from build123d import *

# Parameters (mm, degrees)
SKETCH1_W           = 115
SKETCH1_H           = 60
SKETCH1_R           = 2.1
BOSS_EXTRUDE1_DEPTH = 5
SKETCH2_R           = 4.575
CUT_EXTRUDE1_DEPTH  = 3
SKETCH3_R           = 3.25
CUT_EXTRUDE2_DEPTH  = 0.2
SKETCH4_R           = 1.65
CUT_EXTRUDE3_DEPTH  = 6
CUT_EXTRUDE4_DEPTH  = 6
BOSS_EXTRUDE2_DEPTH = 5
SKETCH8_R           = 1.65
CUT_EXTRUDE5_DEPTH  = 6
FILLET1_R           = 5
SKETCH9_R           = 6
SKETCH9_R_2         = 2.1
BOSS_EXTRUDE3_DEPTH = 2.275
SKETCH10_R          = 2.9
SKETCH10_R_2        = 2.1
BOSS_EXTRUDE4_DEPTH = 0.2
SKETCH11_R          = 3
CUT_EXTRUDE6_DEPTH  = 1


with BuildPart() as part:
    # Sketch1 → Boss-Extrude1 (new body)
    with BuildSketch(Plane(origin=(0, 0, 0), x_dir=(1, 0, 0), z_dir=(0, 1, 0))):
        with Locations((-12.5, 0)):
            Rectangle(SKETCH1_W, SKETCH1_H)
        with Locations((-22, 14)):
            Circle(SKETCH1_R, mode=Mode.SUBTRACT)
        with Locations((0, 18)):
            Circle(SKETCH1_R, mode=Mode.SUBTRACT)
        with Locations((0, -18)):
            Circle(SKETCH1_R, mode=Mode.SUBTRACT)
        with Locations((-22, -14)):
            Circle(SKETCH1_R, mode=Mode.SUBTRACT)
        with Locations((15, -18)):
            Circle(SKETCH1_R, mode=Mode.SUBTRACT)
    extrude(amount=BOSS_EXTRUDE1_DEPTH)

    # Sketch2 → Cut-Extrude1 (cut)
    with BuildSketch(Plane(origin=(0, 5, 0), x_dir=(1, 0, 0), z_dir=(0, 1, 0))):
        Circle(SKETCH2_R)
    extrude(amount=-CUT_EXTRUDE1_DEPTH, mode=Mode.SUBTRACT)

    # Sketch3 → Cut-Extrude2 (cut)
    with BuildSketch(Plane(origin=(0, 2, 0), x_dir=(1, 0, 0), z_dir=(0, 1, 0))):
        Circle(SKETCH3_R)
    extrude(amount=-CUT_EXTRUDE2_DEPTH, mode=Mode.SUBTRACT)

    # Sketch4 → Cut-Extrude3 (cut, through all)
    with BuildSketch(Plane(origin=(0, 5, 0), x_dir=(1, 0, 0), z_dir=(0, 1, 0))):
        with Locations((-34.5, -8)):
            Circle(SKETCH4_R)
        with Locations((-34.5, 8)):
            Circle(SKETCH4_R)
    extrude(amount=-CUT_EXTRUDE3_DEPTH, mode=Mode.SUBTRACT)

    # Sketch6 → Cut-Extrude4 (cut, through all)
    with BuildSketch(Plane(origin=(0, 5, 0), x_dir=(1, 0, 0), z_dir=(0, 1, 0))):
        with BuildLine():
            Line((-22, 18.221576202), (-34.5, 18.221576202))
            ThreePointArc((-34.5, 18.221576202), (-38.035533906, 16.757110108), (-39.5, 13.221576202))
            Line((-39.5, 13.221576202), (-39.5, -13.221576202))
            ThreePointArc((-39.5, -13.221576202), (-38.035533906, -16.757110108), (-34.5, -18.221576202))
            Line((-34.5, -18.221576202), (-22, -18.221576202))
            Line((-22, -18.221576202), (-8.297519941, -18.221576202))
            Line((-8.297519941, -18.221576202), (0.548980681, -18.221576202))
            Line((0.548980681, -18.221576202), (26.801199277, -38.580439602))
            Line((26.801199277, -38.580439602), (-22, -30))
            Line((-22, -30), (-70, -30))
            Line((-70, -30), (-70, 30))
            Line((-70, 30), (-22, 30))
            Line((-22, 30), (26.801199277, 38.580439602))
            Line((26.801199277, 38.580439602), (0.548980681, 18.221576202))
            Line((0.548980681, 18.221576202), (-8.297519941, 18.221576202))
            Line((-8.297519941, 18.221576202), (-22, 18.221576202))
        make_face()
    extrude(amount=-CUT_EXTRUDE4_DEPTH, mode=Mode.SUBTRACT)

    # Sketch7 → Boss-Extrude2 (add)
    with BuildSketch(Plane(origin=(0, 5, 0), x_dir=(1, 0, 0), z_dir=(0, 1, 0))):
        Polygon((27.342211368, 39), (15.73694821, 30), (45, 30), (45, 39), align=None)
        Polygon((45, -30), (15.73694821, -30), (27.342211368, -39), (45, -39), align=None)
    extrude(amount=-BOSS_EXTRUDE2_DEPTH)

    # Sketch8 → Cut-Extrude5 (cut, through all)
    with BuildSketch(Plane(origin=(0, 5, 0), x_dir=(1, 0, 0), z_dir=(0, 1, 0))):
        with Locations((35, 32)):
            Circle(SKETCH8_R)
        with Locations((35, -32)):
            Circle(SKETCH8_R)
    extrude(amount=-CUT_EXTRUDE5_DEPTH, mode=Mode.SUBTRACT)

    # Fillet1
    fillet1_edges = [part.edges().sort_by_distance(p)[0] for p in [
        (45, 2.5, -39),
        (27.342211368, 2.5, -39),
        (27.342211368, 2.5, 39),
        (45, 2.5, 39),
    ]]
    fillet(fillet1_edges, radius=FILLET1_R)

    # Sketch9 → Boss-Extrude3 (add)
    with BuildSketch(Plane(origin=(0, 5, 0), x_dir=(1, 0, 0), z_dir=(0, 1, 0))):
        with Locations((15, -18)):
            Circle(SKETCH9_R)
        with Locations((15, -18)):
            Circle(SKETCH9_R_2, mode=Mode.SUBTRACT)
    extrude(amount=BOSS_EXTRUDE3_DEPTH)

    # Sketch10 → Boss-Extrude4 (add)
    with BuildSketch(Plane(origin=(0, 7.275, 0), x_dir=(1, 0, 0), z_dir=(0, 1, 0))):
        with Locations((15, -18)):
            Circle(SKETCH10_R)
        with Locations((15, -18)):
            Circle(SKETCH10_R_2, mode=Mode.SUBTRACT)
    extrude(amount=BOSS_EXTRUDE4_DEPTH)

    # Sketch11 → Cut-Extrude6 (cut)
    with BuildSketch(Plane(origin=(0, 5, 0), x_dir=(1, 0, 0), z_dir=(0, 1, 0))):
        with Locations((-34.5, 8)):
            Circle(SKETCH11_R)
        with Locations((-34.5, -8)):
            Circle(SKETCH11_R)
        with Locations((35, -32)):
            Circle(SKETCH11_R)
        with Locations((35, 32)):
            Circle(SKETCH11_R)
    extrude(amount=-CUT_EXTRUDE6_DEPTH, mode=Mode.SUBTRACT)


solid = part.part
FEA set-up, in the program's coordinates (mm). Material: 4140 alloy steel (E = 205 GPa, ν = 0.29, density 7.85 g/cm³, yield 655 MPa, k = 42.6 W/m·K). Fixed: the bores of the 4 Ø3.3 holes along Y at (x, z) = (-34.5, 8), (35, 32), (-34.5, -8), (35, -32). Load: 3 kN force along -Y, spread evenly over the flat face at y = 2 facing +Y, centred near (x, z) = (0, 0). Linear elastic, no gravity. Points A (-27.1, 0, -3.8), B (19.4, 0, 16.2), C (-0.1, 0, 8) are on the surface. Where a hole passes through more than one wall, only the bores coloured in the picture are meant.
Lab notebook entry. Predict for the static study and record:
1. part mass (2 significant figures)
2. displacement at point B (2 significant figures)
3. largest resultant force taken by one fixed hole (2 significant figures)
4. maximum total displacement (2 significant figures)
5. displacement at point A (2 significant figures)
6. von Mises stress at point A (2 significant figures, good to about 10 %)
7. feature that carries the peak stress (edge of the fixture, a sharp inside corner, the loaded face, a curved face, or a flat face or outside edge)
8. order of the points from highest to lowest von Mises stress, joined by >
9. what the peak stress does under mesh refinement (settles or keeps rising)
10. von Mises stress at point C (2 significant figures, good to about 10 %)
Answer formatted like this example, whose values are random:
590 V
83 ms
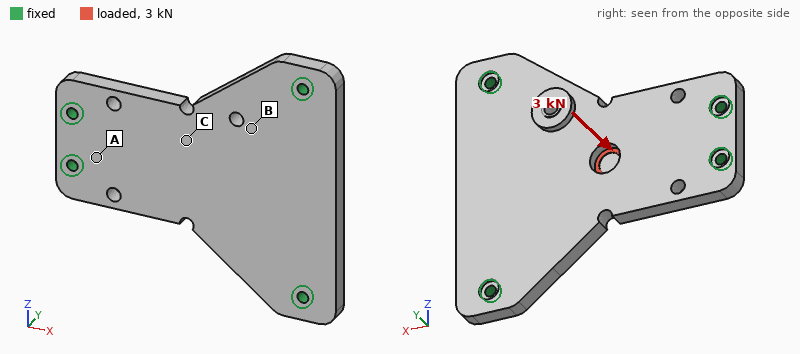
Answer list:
170 g
0.057 mm
810 N
0.11 mm
0.018 mm
99 MPa
edge of the fixture
C > A > B
keeps rising
180 MPa
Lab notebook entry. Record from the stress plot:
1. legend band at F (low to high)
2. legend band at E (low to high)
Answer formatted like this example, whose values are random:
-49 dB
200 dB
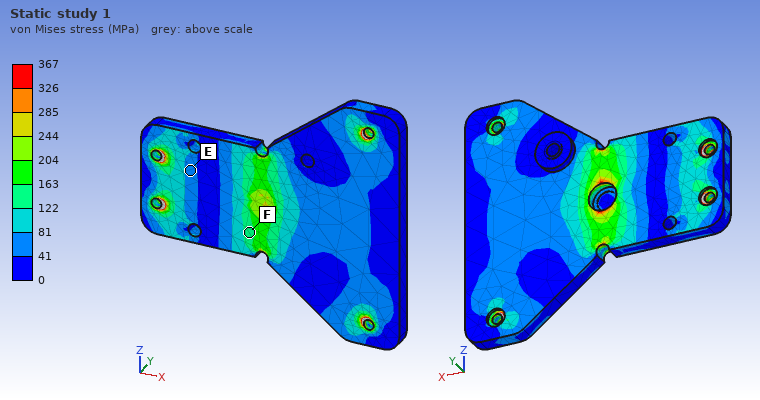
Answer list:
122 to 163 MPa
41 to 81 MPa
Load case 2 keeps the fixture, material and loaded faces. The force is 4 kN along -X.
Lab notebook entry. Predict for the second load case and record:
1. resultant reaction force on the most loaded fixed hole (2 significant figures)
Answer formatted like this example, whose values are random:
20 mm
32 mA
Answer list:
1.2 kN
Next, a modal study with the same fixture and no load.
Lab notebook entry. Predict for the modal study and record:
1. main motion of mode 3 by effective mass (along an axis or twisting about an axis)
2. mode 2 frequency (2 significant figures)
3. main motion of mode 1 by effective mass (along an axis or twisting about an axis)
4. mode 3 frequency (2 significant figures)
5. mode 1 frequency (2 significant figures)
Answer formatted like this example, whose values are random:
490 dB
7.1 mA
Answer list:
twisting about X
6200 Hz
along Y
7200 Hz
3800 Hz
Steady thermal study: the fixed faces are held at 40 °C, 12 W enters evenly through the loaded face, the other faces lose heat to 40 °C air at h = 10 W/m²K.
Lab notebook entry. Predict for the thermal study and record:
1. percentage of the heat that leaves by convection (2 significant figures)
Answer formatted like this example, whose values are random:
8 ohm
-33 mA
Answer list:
9.8 %
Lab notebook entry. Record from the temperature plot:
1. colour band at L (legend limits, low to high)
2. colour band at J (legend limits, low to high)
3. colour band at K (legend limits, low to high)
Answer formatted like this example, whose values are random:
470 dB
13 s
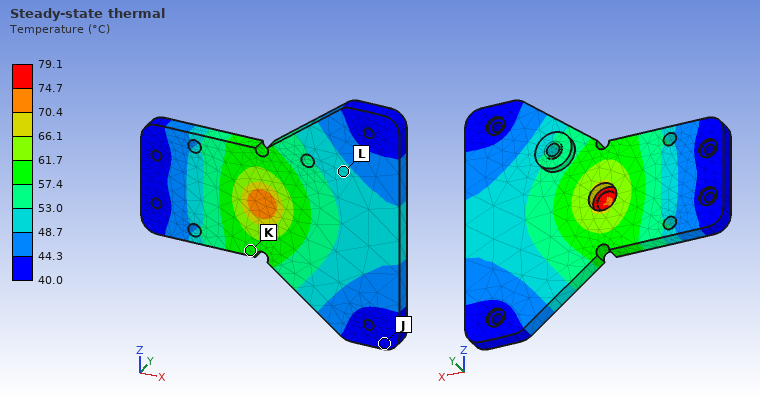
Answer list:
48.7 to 53.0 °C
40.0 to 44.3 °C
57.4 to 61.7 °C
